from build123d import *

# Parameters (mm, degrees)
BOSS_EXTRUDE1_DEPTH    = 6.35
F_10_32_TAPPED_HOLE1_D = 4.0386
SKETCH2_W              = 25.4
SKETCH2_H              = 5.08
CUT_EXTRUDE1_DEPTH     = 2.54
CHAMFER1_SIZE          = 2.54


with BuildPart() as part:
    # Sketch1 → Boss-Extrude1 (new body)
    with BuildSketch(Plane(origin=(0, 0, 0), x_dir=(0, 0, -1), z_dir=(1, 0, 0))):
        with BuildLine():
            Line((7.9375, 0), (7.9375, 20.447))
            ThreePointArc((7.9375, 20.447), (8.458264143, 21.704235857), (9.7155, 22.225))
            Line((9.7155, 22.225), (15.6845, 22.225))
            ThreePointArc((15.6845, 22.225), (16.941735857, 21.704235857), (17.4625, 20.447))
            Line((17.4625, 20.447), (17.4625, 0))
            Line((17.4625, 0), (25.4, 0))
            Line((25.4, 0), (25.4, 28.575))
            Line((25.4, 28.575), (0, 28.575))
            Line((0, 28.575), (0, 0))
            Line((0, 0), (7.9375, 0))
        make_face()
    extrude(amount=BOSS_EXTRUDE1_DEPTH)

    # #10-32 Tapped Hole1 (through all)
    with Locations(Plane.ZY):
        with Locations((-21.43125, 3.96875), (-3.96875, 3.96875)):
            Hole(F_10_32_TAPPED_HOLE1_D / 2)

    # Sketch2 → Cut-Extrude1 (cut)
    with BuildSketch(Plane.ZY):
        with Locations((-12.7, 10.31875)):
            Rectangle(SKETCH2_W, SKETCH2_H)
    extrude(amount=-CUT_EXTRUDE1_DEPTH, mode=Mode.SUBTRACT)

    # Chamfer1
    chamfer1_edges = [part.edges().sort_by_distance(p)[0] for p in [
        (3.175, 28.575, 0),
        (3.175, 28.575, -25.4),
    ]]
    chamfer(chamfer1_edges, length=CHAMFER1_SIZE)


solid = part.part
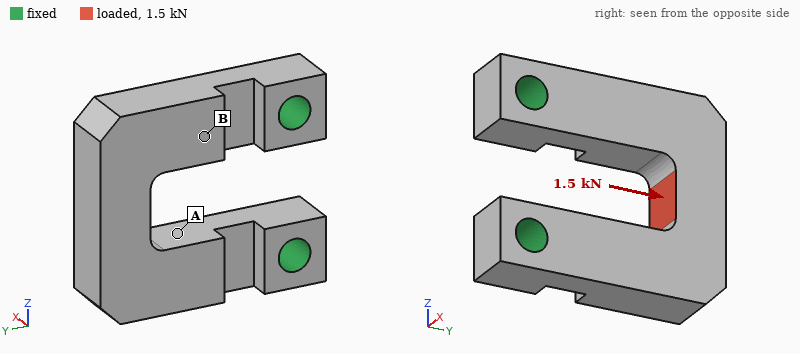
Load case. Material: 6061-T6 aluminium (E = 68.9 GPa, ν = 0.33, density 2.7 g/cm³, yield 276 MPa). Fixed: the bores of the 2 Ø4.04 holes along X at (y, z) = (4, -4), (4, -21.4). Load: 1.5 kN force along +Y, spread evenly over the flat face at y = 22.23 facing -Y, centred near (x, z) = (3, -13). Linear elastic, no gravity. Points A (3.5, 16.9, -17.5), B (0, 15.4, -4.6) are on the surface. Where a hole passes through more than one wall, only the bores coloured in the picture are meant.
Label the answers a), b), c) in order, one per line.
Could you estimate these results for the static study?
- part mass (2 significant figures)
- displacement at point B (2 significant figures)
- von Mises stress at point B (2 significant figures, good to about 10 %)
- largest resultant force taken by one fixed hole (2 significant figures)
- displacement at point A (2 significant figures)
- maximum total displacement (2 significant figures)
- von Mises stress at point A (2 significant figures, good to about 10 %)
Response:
a) 7.7 g
b) 22 µm
c) 14 MPa
d) 770 N
e) 21 µm
f) 59 µm
g) 43 MPa
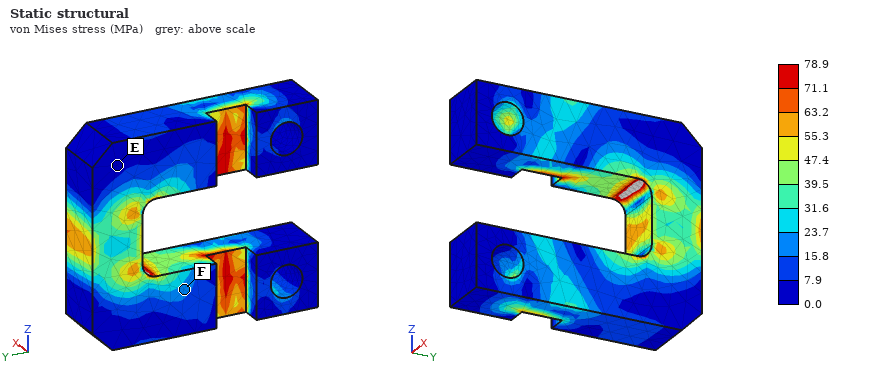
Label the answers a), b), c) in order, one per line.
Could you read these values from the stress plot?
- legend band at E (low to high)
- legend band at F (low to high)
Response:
a) 0.0 to 7.9 MPa
b) 15.8 to 23.7 MPa
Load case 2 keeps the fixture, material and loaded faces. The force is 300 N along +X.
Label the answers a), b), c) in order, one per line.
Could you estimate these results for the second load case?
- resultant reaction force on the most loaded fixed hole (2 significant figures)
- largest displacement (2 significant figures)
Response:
a) 150 N
b) 0.12 mm
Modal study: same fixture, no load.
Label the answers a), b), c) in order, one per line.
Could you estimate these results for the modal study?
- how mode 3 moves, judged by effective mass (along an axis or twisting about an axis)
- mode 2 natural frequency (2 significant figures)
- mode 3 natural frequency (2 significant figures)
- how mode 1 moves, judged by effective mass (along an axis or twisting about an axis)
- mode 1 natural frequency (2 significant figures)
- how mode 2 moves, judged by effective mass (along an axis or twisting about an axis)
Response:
a) along Z
b) 11 kHz
c) 12 kHz
d) along X
e) 4300 Hz
f) along Z
